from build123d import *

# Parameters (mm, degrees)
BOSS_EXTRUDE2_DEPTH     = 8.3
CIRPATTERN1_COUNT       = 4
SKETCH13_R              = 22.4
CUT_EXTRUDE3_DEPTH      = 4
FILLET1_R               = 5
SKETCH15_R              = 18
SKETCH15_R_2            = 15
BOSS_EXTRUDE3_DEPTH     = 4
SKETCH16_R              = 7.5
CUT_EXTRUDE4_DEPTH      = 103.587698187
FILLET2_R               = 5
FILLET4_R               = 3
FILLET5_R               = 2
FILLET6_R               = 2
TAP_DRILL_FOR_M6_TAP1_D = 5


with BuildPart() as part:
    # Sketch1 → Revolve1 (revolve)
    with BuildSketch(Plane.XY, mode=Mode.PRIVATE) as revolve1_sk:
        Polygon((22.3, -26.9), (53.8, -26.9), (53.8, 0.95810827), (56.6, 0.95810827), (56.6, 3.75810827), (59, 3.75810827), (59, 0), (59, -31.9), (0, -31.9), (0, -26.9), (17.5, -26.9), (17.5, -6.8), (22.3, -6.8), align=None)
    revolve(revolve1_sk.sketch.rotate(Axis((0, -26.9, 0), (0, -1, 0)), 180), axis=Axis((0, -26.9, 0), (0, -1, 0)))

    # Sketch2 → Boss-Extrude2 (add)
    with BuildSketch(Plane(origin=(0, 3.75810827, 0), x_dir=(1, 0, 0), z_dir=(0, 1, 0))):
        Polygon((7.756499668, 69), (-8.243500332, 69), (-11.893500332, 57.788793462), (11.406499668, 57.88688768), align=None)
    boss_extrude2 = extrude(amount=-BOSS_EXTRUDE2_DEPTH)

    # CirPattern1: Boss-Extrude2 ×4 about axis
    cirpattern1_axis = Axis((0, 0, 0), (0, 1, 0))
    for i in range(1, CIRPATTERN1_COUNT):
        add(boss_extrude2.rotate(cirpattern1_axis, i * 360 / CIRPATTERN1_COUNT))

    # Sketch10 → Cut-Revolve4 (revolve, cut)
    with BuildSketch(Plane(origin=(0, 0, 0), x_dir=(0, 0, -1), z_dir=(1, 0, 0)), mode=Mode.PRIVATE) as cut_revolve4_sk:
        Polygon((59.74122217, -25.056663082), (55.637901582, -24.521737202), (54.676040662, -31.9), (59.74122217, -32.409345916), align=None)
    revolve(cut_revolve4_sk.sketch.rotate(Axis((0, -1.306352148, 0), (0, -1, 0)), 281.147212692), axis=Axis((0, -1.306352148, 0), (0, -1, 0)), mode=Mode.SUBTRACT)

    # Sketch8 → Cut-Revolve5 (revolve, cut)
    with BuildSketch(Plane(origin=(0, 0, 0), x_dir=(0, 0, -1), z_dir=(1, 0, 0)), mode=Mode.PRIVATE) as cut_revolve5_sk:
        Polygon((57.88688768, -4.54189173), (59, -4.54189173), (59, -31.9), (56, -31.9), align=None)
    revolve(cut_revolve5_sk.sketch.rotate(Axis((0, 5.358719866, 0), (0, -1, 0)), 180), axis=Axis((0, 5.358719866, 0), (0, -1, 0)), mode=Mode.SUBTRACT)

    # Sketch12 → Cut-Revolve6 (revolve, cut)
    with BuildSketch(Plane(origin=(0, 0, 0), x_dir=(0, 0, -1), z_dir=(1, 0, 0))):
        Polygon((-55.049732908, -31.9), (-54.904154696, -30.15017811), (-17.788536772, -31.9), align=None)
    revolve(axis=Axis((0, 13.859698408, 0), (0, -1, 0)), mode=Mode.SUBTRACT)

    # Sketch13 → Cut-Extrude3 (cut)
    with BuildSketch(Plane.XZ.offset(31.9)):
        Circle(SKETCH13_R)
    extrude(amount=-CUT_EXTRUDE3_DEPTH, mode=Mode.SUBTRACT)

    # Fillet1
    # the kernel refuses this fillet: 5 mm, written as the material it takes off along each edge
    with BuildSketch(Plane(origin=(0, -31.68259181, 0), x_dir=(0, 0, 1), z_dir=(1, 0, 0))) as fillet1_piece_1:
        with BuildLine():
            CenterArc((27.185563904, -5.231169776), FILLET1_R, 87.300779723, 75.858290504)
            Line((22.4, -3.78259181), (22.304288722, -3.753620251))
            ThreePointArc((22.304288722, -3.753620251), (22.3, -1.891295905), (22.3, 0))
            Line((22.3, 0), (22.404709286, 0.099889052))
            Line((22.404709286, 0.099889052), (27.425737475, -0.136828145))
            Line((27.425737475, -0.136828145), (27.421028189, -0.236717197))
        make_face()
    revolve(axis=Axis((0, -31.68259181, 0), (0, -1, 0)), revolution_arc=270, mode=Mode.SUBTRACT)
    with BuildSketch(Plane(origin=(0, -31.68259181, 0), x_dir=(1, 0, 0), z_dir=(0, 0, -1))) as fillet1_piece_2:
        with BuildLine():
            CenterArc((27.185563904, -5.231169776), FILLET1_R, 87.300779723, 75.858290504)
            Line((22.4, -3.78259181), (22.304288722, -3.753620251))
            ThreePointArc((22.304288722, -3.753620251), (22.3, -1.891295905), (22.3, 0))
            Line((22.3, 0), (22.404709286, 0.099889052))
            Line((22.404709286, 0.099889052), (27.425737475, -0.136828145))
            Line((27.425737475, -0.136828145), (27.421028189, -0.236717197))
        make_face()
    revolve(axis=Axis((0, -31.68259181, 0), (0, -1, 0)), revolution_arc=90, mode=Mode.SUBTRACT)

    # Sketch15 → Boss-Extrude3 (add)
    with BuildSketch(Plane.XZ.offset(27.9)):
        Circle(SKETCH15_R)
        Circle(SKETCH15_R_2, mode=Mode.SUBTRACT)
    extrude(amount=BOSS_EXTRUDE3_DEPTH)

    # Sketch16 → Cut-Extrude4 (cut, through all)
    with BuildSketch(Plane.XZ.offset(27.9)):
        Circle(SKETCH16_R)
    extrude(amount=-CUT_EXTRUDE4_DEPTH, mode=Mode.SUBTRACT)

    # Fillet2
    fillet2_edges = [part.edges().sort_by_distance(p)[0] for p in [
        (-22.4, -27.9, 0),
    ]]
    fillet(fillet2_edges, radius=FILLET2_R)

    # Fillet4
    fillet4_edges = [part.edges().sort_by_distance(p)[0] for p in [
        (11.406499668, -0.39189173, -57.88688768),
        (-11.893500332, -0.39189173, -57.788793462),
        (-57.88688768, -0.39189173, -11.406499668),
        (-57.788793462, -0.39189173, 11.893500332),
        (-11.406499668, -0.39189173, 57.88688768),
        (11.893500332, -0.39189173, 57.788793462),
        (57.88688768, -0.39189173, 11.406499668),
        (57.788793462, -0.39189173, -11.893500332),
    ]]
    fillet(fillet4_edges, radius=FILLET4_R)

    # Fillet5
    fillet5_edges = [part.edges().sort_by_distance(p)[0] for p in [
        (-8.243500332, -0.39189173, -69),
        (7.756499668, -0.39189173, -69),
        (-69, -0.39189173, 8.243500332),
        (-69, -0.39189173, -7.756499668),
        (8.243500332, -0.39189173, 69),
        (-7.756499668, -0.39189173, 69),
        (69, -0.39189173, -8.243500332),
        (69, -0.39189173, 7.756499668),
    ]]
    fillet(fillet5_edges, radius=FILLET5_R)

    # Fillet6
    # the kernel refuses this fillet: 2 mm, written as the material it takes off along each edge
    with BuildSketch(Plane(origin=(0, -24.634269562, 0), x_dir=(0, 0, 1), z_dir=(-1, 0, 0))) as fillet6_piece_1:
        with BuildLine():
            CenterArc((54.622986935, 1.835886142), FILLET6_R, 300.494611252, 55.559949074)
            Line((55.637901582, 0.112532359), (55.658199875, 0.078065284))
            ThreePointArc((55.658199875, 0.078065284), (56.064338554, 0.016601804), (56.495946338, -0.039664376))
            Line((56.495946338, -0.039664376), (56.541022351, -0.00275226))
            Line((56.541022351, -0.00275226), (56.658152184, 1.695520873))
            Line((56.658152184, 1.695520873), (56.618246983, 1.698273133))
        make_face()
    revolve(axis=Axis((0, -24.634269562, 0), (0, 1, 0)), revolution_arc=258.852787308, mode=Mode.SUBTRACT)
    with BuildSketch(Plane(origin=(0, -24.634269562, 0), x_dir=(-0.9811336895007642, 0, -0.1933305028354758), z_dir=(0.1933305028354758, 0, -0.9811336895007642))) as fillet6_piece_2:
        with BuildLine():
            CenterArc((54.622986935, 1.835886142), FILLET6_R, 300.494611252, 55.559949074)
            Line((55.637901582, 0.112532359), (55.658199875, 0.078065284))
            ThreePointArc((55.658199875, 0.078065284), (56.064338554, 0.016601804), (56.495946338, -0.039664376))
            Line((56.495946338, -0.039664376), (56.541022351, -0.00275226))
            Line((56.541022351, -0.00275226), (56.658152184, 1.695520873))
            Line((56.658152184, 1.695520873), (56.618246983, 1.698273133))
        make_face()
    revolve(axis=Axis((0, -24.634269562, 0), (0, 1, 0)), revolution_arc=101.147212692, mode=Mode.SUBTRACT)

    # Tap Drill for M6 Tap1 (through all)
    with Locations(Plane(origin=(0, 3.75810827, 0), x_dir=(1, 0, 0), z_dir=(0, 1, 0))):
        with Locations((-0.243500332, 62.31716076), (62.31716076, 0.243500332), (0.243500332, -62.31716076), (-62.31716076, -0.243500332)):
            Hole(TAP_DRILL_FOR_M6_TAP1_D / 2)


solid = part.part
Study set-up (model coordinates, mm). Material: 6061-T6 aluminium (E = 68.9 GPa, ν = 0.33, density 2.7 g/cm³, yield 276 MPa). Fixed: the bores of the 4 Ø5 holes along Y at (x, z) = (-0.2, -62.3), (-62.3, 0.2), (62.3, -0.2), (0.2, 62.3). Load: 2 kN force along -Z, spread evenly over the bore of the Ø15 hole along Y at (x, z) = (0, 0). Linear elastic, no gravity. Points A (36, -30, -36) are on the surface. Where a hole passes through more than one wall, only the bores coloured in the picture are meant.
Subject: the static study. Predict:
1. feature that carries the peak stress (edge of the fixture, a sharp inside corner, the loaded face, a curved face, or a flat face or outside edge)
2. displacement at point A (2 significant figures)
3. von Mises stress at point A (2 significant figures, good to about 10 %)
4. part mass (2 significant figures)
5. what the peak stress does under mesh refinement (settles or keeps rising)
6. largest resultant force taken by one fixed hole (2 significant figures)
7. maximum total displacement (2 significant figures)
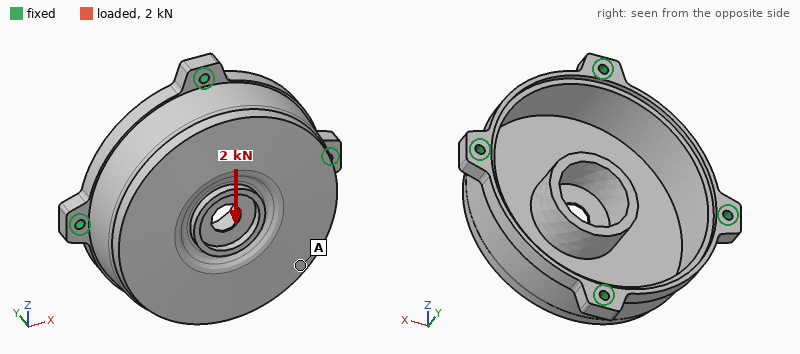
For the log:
a sharp inside corner
11 µm
5.1 MPa
240 g
keeps rising
700 N
22 µm
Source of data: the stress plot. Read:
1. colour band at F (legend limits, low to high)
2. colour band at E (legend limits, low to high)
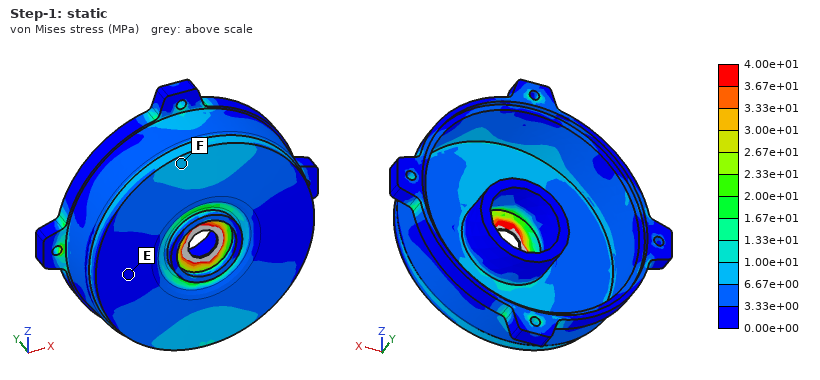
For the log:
6.67e+00 to 1.00e+01 MPa
0.00e+00 to 3.33e+00 MPa
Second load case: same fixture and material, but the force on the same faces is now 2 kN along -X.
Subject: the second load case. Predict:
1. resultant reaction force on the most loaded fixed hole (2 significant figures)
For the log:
700 N
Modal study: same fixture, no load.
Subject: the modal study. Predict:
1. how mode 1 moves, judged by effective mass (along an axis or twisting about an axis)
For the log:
along Y
